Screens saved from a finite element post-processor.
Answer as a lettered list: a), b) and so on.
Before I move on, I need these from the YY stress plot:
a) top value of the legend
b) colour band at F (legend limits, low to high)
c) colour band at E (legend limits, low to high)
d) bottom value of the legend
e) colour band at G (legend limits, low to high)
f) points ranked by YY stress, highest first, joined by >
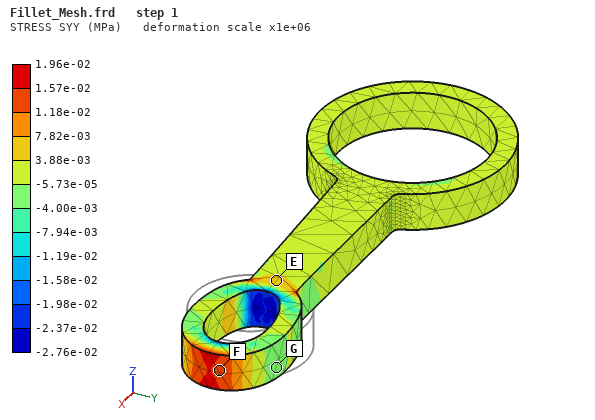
a) 1.96e-02 MPa
b) 1.18e-02 to 1.57e-02 MPa
c) 3.88e-03 to 7.82e-03 MPa
d) -2.76e-02 MPa
e) -4.00e-03 to -5.73e-05 MPa
f) F > E > G
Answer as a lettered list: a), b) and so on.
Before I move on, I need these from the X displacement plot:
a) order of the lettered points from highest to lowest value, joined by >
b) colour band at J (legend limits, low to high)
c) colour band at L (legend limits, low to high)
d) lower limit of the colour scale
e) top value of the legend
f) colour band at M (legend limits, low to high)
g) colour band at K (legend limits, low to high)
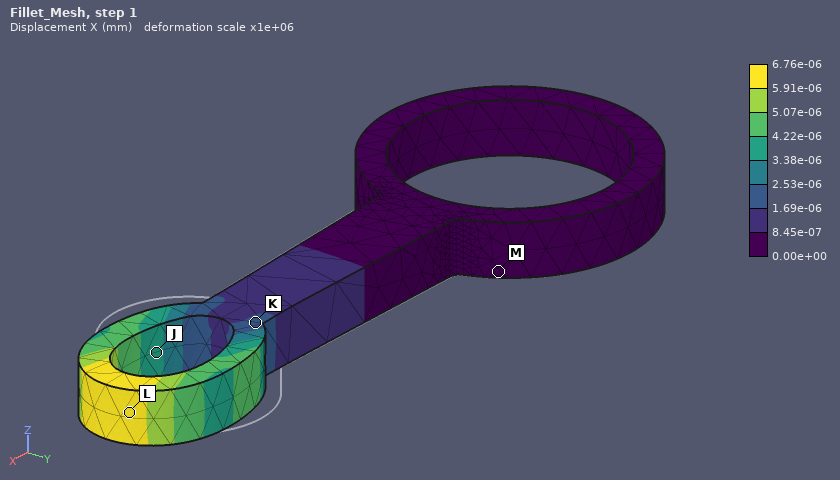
a) L > J > K > M
b) 3.38e-06 to 4.22e-06 mm
c) 5.91e-06 to 6.76e-06 mm
d) 0.00e+00 mm
e) 6.76e-06 mm
f) 0.00e+00 to 8.45e-07 mm
g) 1.69e-06 to 2.53e-06 mm
